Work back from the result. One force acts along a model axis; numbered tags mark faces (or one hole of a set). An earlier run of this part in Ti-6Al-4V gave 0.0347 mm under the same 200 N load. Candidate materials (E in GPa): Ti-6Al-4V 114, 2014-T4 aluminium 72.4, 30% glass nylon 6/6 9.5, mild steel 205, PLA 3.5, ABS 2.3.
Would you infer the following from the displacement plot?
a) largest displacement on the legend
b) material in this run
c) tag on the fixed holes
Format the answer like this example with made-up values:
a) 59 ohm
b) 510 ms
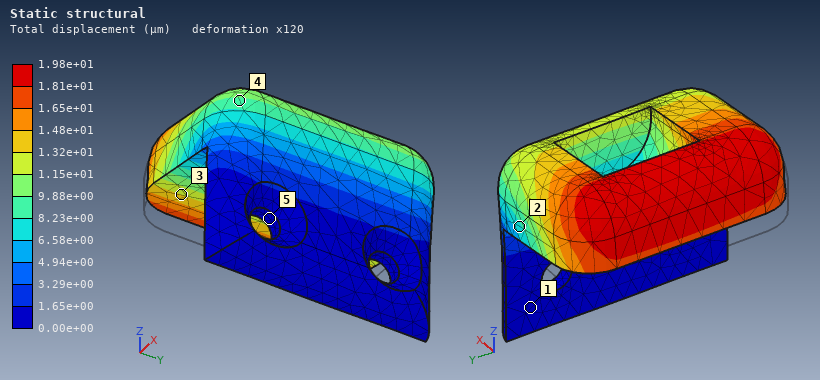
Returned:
a) 1.98e+01 µm
b) mild steel
c) 5
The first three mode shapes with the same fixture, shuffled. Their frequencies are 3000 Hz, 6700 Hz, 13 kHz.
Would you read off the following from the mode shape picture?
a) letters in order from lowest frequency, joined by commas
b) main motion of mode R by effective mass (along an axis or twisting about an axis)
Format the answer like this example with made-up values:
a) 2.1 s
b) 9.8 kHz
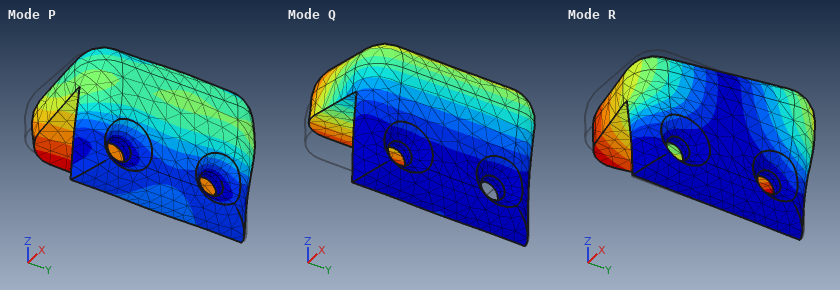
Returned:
a) Q, R, P
b) along Y
